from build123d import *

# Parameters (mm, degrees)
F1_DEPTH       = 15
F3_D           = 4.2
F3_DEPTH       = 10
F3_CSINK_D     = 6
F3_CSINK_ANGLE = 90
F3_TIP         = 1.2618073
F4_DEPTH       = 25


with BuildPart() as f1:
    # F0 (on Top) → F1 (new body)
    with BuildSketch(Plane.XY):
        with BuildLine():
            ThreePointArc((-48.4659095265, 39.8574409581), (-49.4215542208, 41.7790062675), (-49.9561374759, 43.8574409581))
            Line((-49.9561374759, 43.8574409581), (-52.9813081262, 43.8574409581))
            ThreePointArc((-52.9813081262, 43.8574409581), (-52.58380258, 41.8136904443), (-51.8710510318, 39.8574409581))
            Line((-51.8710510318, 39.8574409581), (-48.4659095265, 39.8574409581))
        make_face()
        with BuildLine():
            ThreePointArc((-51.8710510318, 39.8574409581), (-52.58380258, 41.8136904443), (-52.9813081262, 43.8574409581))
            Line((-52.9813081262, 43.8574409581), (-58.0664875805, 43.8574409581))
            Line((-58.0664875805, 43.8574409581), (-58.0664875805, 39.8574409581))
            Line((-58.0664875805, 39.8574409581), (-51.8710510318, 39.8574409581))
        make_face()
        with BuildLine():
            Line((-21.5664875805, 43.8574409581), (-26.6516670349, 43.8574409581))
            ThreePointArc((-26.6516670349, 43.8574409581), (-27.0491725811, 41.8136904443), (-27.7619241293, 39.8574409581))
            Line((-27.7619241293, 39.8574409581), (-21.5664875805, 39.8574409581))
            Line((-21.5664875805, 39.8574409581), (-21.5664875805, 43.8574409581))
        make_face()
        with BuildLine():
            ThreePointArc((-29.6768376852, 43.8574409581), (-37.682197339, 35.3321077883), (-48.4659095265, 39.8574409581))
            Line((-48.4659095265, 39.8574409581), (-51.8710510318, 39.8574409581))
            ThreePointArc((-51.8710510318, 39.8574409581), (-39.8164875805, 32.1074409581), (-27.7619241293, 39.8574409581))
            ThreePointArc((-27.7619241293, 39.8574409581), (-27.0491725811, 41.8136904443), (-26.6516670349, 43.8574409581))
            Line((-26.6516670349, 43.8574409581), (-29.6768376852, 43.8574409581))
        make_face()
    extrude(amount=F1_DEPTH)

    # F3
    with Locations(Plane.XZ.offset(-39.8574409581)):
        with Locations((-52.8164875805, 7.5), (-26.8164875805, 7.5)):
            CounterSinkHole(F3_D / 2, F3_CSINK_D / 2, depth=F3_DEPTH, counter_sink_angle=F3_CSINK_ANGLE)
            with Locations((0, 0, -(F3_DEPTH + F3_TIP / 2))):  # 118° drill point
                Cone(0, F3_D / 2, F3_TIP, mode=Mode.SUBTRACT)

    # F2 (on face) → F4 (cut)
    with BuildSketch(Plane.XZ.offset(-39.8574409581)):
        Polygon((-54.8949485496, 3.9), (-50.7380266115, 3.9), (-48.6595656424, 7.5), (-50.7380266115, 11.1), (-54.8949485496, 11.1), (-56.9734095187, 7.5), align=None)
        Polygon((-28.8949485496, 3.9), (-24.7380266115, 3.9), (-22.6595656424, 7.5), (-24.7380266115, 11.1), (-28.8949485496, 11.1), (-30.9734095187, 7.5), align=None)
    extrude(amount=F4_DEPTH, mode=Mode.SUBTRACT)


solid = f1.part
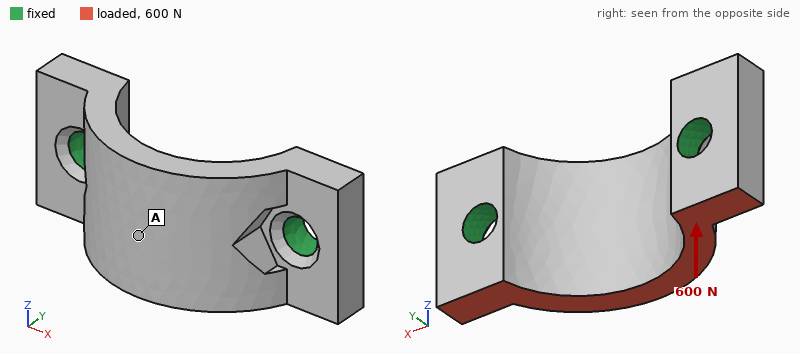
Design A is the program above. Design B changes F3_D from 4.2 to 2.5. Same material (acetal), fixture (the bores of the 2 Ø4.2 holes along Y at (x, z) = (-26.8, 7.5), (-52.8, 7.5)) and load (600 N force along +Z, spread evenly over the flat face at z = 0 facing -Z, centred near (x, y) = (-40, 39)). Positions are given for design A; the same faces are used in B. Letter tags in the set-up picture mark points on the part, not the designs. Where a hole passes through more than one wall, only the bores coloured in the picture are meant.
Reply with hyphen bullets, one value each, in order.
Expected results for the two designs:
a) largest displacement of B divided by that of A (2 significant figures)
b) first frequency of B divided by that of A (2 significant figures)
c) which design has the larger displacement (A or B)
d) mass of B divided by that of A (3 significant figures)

- 2.7
- 0.58
- B
- 1.02
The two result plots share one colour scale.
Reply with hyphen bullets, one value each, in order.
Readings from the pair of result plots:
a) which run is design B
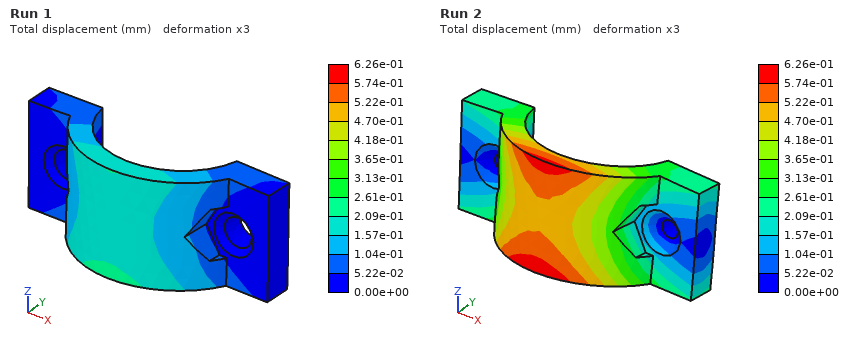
- Run 2
